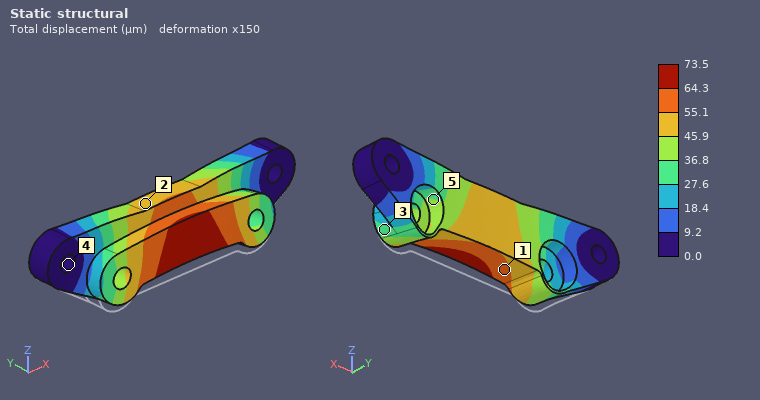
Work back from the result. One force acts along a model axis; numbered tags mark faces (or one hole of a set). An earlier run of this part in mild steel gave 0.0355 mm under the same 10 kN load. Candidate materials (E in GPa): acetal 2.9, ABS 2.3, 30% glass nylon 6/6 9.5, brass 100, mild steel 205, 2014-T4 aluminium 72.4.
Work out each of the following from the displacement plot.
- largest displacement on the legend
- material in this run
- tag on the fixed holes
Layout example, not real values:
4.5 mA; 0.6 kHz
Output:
73.5 µm; brass; 4
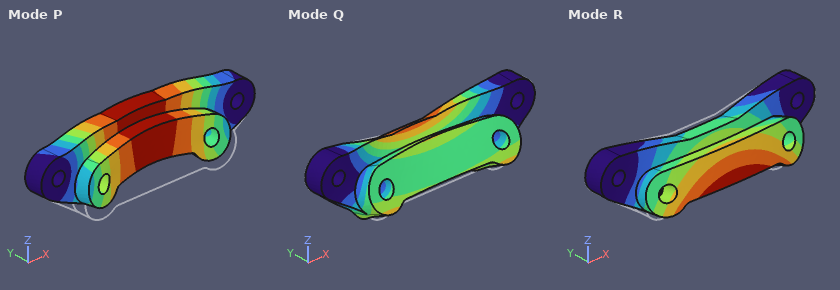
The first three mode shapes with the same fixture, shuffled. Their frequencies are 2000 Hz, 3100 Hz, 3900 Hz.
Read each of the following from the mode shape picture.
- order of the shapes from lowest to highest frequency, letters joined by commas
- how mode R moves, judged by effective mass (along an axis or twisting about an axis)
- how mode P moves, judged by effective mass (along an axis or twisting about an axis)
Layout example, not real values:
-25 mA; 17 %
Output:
R, P, Q; along Y; along Z
